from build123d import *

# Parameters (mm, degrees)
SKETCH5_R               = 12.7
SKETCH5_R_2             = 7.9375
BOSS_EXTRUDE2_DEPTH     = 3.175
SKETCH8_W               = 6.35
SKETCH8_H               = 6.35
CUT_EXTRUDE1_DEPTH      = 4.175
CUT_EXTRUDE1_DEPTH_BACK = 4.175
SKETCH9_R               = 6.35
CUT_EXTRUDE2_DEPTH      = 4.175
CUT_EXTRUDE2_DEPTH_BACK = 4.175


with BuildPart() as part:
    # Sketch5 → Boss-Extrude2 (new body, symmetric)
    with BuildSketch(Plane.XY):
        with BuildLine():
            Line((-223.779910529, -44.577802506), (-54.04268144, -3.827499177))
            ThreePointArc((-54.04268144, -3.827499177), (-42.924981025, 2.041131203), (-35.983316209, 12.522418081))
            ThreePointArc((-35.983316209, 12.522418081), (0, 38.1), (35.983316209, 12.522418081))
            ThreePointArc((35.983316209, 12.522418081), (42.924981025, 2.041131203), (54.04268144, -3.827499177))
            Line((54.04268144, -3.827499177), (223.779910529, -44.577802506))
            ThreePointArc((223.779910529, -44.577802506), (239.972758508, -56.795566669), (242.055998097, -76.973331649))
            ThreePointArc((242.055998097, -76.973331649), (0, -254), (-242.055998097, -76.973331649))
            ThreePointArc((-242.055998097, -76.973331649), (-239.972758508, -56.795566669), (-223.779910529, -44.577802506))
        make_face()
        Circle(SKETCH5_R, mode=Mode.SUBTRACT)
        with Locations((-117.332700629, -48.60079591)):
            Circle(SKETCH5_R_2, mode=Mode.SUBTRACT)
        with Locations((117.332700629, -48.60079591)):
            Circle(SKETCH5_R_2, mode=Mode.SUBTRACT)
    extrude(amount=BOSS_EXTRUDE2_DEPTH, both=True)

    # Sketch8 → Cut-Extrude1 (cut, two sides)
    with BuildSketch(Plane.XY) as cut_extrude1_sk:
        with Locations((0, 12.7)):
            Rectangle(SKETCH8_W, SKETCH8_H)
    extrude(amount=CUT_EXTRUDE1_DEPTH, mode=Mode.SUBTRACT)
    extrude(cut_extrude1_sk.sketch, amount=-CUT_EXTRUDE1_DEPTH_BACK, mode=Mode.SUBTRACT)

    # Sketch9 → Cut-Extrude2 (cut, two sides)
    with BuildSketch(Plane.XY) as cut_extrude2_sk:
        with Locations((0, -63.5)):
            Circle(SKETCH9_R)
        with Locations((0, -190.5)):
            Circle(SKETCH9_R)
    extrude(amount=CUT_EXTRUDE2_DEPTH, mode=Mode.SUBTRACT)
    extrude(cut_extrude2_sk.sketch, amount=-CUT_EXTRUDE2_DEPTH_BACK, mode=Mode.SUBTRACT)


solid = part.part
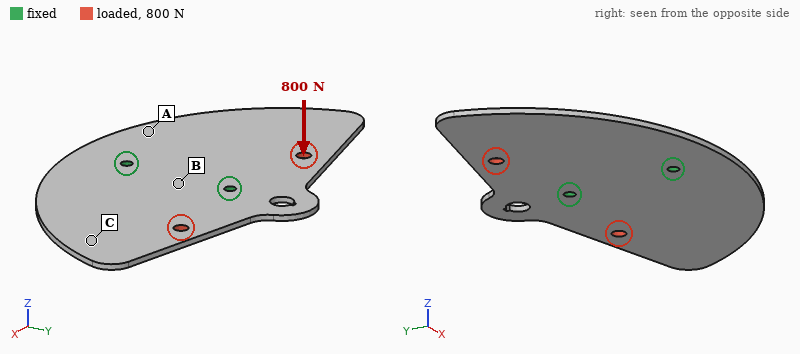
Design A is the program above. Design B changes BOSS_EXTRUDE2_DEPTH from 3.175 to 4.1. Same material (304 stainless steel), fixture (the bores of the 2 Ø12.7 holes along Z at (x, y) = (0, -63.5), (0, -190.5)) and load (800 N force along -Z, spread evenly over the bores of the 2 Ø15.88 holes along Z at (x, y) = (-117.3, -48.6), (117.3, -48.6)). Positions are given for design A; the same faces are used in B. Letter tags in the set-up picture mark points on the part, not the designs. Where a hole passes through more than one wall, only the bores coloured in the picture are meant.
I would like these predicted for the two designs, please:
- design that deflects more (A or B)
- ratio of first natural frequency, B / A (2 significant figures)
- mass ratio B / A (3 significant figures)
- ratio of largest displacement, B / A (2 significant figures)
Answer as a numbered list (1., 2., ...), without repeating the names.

1. A
2. 1.3
3. 1.29
4. 0.47
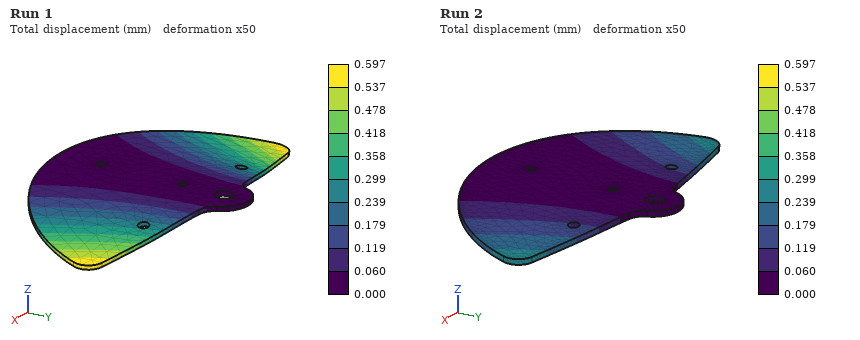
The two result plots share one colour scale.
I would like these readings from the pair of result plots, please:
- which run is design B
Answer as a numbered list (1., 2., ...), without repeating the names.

1. Run 2
